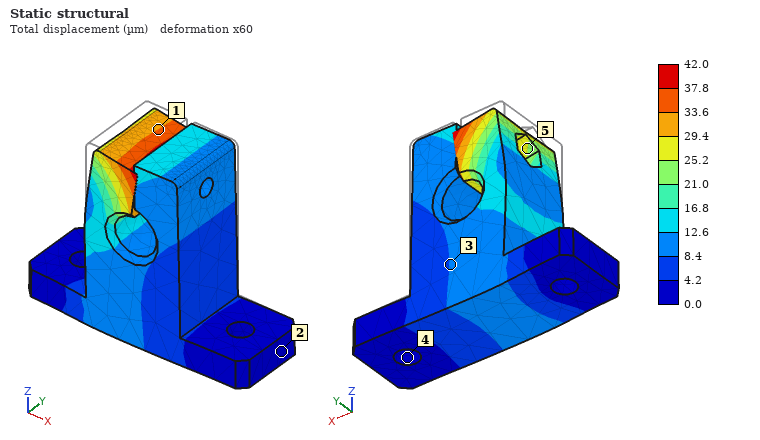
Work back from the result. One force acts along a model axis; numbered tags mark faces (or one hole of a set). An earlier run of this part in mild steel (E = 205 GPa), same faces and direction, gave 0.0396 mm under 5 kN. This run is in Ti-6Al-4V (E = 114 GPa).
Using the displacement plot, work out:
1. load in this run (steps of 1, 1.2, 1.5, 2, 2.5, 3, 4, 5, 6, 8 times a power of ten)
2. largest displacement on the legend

3 kN
42.0 µm
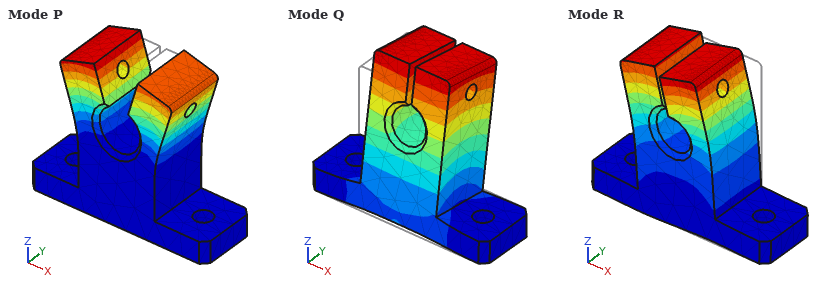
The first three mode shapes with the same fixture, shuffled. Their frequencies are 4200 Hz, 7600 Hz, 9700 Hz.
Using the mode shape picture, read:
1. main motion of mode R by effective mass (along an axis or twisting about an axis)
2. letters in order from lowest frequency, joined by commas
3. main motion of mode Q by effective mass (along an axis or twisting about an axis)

along X
Q, R, P
along Y
